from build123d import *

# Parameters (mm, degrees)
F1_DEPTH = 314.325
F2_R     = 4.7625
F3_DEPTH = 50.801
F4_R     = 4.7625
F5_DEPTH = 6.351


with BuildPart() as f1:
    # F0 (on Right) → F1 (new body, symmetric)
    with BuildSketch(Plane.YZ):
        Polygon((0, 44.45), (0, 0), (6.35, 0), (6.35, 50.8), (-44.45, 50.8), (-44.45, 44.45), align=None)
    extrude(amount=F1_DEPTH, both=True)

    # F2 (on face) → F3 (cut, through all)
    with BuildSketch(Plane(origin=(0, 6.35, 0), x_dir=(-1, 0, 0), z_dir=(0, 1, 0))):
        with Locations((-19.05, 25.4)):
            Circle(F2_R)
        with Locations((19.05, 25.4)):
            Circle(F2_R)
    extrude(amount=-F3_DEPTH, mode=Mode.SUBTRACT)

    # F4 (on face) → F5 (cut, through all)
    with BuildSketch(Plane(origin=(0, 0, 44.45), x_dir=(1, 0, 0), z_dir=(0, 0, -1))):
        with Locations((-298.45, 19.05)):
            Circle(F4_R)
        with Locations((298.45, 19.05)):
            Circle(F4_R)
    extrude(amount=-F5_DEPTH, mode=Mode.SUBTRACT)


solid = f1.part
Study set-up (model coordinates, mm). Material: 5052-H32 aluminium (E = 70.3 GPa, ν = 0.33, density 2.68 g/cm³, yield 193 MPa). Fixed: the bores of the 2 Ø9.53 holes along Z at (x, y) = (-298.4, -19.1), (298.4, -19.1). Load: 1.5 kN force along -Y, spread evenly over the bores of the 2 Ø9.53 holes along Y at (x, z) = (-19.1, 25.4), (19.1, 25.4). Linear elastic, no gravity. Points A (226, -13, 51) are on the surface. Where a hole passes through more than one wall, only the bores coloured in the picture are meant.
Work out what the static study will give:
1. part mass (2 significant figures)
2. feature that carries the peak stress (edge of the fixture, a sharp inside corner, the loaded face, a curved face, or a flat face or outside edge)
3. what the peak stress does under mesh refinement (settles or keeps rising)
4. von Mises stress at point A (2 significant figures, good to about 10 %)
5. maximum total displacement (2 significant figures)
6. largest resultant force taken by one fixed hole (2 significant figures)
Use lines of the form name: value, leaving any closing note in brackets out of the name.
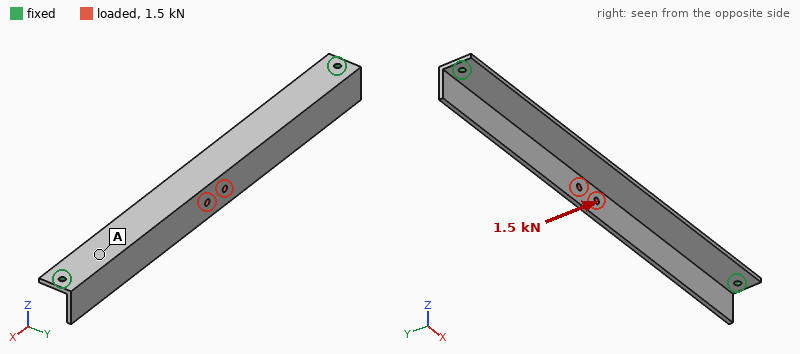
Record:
part mass: 1.0 kg
feature that carries the peak stress: edge of the fixture
what the peak stress does under mesh refinement: keeps rising
von Mises stress at point A: 18 MPa
maximum total displacement: 1.7 mm
largest resultant force taken by one fixed hole: 870 N
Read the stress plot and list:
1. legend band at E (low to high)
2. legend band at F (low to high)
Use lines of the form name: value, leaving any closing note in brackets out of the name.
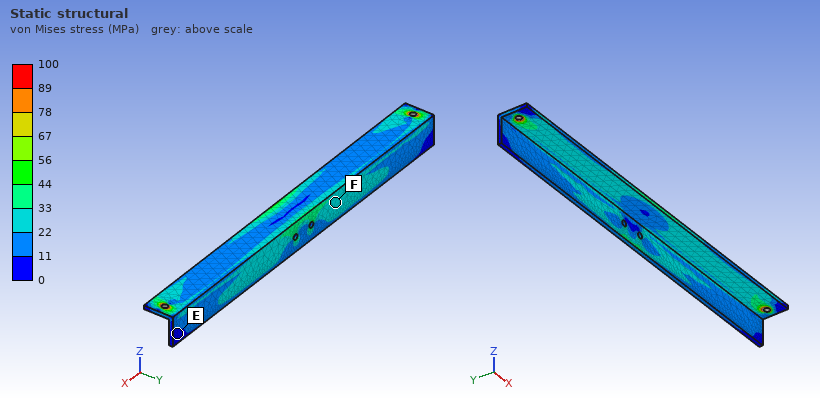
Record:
legend band at E: 0 to 11 MPa
legend band at F: 22 to 33 MPa
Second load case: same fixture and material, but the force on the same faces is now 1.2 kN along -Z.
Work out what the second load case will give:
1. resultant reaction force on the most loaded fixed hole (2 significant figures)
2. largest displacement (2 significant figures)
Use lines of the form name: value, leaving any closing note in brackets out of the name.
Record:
resultant reaction force on the most loaded fixed hole: 2.1 kN
largest displacement: 0.65 mm
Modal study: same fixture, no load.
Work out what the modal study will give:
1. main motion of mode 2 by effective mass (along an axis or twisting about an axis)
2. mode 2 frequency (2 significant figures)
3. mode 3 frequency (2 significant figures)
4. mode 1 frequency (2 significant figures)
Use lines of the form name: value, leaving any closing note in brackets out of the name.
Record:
main motion of mode 2 by effective mass: along Z
mode 2 frequency: 330 Hz
mode 3 frequency: 670 Hz
mode 1 frequency: 310 Hz
